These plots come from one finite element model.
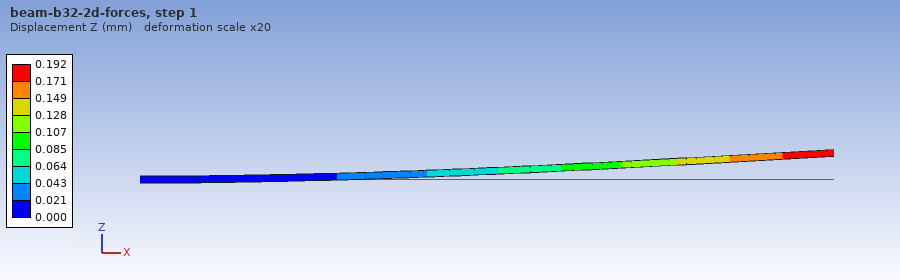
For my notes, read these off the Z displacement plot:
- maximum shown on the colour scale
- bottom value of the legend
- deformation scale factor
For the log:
0.192 mm
0.000 mm
20
